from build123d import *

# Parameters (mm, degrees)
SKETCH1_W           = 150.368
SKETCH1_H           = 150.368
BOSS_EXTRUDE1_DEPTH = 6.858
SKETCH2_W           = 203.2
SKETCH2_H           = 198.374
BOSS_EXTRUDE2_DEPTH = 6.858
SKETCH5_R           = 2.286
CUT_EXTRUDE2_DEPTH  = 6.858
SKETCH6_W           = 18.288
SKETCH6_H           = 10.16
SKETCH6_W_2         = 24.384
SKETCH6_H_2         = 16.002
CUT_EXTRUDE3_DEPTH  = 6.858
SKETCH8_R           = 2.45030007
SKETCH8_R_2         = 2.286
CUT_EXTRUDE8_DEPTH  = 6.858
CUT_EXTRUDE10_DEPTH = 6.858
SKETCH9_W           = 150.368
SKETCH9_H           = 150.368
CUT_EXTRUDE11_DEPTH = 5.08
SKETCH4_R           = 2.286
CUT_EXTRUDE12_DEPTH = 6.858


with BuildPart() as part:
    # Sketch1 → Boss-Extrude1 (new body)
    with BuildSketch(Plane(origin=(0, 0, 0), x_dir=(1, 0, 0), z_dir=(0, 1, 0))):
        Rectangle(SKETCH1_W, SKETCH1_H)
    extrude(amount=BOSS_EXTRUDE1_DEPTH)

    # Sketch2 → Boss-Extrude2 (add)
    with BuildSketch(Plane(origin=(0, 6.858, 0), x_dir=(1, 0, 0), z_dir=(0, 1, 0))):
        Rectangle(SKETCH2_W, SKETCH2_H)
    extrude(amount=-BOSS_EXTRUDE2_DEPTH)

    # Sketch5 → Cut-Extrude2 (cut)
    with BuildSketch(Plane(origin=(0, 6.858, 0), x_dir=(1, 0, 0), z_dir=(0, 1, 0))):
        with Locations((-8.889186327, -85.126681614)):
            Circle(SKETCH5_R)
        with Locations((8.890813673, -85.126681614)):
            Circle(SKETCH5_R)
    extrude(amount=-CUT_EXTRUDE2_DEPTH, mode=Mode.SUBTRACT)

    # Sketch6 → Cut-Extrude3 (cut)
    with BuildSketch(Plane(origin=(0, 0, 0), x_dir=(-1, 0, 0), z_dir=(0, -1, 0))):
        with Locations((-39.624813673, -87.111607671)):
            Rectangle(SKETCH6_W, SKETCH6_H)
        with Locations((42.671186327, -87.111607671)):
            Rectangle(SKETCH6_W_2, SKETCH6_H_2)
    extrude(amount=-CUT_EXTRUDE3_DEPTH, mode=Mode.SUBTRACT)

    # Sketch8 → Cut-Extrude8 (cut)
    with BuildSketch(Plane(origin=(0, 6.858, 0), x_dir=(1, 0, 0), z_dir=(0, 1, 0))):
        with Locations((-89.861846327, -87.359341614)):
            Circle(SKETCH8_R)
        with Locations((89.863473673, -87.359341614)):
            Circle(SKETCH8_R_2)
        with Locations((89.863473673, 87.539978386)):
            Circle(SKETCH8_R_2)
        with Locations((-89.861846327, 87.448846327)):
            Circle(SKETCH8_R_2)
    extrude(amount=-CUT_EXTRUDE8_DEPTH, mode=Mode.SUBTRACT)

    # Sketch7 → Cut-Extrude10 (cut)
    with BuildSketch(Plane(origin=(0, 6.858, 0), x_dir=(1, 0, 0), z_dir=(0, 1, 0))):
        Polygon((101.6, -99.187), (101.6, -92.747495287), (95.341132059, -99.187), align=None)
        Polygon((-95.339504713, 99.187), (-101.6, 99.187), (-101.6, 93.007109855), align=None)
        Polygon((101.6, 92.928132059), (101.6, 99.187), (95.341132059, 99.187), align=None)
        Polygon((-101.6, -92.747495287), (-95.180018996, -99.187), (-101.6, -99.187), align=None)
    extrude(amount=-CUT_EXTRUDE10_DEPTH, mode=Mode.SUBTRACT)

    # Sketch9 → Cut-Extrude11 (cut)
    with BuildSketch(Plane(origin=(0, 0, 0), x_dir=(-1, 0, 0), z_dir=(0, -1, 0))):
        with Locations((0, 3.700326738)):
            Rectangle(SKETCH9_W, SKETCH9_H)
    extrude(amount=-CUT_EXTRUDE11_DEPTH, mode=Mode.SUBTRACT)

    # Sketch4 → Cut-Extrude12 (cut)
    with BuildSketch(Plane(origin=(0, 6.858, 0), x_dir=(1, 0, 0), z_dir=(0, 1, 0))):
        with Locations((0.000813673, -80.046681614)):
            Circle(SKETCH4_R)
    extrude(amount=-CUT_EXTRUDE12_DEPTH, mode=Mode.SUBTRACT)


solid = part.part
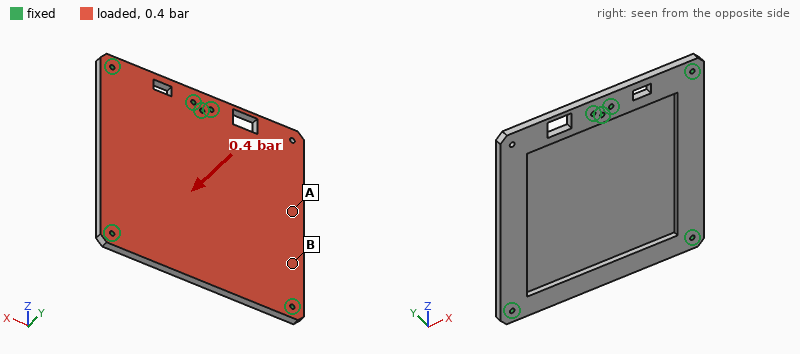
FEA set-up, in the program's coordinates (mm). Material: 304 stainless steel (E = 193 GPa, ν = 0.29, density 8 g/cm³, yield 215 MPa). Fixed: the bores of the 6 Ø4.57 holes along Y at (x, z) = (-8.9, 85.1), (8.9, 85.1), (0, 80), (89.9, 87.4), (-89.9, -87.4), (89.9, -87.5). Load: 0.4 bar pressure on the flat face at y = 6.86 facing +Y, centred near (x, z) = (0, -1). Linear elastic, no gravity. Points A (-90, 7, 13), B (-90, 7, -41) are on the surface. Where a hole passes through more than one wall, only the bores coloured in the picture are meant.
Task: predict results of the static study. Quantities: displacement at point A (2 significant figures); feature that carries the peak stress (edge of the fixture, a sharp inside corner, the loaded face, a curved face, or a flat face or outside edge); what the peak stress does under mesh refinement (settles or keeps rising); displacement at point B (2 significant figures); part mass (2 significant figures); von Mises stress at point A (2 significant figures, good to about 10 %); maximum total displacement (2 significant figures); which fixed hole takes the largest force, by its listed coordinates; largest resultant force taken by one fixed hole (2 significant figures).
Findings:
0.12 mm
edge of the fixture
keeps rising
0.054 mm
1.3 kg
24 MPa
0.35 mm
(-89.9, -87.4)
1.0 kN
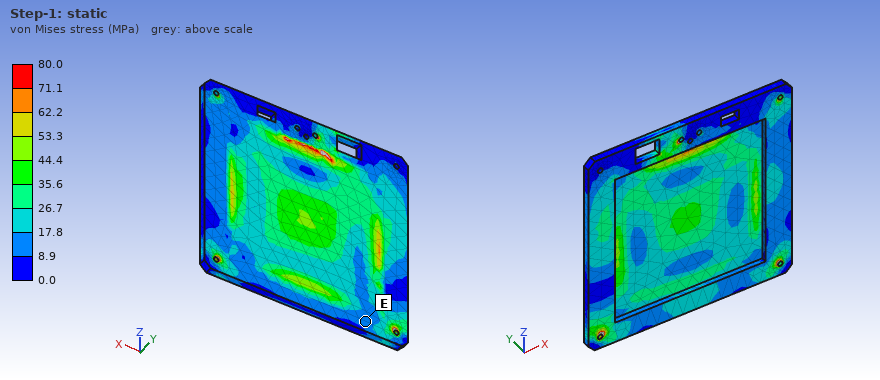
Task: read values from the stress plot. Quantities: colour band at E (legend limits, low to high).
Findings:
8.9 to 17.8 MPa
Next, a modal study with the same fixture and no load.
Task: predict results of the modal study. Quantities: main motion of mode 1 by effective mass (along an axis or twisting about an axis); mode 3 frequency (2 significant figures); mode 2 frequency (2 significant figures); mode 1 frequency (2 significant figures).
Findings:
along Y
970 Hz
590 Hz
500 Hz
